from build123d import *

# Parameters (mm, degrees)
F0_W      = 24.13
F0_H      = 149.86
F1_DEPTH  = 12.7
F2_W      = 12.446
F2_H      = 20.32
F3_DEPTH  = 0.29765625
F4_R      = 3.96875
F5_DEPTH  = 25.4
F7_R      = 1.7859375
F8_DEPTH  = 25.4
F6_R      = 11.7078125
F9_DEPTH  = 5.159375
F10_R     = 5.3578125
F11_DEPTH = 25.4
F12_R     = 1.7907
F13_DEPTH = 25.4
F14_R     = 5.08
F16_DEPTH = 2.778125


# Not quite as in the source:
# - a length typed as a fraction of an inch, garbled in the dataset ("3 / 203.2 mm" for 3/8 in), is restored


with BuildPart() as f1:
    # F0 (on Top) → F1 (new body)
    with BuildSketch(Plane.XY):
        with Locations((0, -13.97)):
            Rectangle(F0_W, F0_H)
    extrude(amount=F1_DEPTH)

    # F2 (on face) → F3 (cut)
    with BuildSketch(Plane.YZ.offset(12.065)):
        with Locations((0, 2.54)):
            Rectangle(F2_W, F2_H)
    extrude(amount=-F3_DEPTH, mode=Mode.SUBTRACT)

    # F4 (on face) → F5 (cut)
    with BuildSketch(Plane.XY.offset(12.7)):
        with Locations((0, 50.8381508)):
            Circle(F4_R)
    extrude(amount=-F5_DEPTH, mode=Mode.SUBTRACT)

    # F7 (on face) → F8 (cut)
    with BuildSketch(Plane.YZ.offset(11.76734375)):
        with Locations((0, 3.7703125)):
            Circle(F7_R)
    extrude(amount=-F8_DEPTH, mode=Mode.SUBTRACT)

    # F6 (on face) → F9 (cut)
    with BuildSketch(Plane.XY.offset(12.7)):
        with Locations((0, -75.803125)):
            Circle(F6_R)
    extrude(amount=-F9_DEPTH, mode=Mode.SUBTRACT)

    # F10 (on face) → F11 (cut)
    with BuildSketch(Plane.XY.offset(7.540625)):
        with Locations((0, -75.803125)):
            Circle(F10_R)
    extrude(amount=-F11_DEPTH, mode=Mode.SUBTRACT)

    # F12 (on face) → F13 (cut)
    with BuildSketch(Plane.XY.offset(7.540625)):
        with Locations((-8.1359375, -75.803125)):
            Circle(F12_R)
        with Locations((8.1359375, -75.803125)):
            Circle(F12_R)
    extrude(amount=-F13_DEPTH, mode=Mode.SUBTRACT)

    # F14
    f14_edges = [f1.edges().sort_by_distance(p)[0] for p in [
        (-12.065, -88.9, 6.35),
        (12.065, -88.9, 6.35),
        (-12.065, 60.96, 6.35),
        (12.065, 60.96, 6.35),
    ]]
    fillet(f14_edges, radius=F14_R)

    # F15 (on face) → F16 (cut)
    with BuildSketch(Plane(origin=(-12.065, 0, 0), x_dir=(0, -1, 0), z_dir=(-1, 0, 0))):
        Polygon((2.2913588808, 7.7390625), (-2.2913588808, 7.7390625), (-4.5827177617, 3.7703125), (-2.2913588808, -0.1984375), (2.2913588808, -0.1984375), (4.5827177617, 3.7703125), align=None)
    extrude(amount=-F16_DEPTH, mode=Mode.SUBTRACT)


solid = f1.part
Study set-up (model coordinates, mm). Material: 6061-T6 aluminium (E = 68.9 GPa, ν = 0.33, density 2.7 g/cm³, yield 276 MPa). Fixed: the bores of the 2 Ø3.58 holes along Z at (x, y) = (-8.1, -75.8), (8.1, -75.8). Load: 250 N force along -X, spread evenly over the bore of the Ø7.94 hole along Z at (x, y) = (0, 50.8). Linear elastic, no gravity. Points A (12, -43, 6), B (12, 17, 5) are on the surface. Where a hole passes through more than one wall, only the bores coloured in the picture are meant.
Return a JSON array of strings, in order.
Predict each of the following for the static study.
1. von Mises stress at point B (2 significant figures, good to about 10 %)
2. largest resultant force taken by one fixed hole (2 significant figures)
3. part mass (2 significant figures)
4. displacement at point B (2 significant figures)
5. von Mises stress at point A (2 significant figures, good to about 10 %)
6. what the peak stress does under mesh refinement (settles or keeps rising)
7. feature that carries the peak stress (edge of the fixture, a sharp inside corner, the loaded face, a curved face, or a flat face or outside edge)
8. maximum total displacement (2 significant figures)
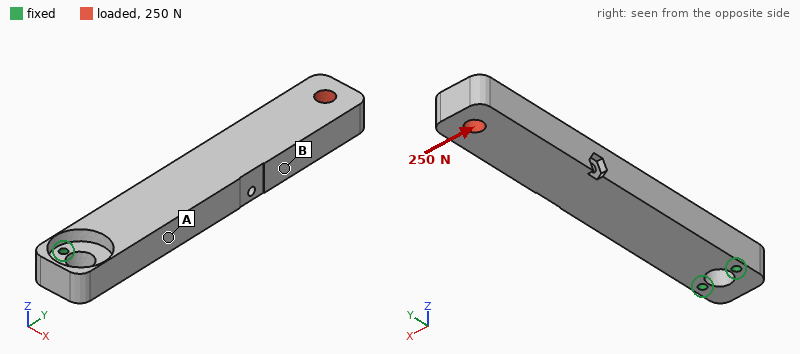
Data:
["6.9 MPa", "1.8 kN", "110 g", "0.13 mm", "19 MPa", "keeps rising", "edge of the fixture", "0.23 mm"]
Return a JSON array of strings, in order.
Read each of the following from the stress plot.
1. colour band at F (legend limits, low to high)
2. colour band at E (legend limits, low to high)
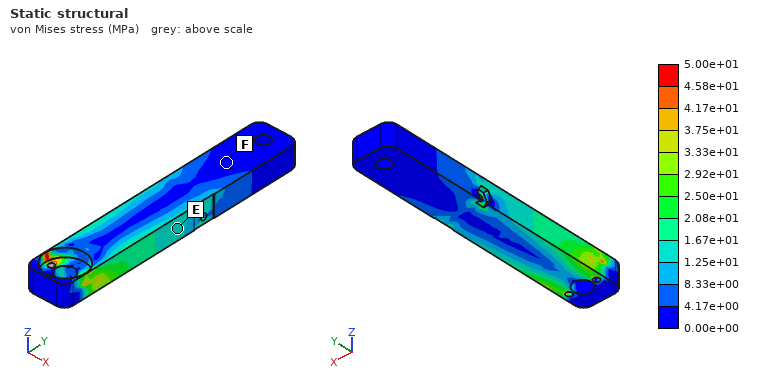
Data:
["0.00e+00 to 4.17e+00 MPa", "1.25e+01 to 1.67e+01 MPa"]
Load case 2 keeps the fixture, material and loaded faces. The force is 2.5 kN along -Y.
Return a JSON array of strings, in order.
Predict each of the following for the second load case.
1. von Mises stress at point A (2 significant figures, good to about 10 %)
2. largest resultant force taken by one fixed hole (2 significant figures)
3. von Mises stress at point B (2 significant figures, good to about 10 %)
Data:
["8.2 MPa", "1.3 kN", "8.1 MPa"]
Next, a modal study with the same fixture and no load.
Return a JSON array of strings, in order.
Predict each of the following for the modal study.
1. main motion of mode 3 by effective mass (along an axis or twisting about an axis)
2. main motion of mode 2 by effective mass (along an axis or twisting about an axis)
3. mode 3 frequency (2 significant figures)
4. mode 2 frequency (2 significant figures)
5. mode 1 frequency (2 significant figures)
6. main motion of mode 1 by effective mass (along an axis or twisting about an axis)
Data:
["along Z", "along X", "2800 Hz", "970 Hz", "400 Hz", "along Z"]
